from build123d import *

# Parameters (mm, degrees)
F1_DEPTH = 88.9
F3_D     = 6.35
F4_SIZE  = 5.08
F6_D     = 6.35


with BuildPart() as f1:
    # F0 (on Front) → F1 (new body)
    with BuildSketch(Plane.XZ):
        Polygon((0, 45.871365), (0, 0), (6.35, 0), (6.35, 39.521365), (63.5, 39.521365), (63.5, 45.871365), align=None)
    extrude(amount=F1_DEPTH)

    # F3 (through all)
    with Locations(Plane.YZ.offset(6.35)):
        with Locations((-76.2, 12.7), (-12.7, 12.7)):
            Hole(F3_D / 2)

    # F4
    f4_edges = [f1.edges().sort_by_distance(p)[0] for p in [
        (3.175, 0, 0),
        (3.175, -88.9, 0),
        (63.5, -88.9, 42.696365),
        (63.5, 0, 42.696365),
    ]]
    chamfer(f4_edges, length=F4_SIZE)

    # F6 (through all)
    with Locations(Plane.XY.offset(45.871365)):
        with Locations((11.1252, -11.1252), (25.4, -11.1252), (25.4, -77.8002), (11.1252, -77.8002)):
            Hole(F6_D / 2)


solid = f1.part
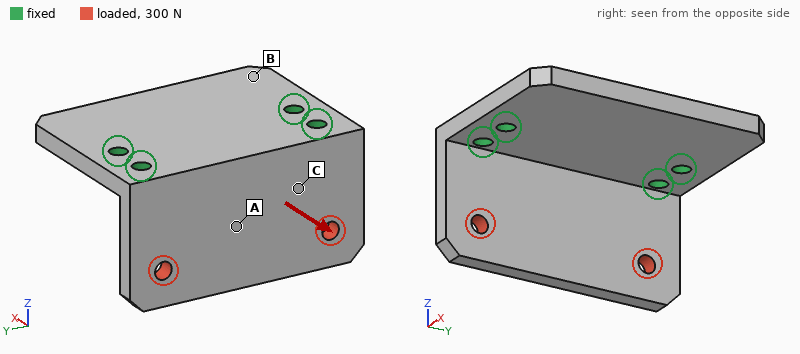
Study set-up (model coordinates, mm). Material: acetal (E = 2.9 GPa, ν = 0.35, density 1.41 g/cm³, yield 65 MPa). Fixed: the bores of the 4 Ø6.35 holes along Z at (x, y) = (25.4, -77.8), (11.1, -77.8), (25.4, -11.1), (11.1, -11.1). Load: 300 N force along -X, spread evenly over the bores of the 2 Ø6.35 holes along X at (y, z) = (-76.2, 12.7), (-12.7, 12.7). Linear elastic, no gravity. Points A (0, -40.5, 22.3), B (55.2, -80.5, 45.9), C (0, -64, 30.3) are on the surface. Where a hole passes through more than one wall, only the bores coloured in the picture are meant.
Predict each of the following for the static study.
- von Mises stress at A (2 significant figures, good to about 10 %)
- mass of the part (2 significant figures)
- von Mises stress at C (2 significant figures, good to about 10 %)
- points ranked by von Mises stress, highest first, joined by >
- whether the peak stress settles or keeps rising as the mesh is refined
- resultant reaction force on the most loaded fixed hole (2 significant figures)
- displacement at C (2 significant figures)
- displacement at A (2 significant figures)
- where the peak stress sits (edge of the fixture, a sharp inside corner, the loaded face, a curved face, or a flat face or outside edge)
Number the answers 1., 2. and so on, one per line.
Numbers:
1. 4.4 MPa
2. 80 g
3. 7.6 MPa
4. C > A > B
5. keeps rising
6. 160 N
7. 0.29 mm
8. 0.48 mm
9. edge of the fixture
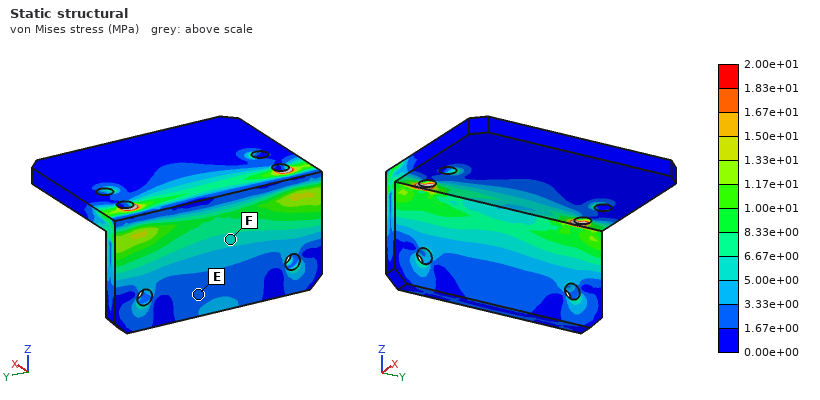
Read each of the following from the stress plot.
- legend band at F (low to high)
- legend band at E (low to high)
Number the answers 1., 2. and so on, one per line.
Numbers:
1. 5.00e+00 to 6.67e+00 MPa
2. 1.67e+00 to 3.33e+00 MPa
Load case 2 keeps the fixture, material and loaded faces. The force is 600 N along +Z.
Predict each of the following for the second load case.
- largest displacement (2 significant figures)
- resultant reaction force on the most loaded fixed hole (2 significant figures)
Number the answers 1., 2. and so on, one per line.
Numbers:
1. 0.20 mm
2. 330 N
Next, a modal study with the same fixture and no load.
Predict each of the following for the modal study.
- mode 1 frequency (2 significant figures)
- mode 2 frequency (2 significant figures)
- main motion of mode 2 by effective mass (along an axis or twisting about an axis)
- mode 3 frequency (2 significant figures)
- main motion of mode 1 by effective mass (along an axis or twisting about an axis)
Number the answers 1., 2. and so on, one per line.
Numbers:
1. 640 Hz
2. 870 Hz
3. along Z
4. 1100 Hz
5. along X
